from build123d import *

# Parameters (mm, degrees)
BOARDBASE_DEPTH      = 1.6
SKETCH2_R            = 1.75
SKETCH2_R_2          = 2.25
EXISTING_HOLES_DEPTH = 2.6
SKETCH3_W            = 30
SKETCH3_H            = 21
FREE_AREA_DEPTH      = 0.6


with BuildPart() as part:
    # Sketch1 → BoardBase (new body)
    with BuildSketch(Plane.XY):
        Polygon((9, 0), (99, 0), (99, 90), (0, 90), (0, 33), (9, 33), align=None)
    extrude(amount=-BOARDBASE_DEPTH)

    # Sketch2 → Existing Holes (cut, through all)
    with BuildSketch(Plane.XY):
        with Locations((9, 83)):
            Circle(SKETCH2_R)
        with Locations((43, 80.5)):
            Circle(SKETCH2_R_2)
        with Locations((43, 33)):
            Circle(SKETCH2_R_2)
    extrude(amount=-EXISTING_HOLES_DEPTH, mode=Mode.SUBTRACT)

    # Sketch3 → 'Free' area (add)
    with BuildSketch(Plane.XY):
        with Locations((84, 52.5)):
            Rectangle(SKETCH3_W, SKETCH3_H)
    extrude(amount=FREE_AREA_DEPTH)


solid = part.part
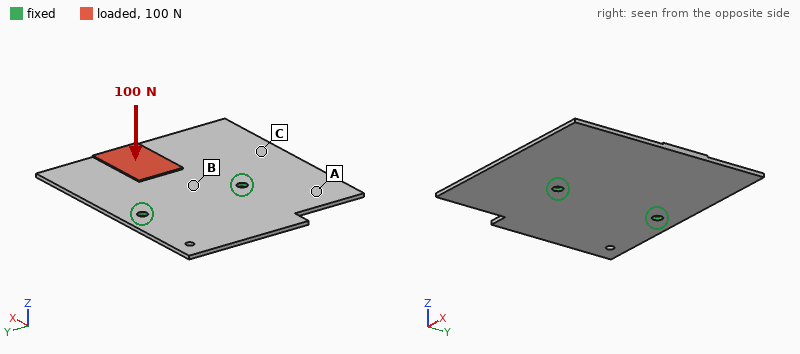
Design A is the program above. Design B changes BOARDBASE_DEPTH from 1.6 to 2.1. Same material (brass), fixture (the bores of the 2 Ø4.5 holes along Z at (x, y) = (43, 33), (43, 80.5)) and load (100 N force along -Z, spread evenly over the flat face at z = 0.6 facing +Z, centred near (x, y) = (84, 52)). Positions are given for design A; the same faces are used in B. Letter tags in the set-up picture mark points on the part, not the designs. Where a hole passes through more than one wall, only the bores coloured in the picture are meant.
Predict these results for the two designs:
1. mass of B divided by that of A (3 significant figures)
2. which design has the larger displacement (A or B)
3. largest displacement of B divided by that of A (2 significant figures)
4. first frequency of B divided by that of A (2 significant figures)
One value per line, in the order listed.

1.30
A
0.45
1.3
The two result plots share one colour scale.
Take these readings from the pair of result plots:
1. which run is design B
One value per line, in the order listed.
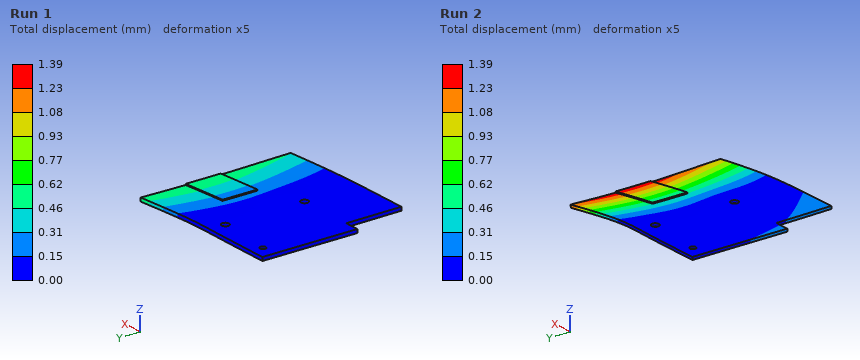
Run 1
